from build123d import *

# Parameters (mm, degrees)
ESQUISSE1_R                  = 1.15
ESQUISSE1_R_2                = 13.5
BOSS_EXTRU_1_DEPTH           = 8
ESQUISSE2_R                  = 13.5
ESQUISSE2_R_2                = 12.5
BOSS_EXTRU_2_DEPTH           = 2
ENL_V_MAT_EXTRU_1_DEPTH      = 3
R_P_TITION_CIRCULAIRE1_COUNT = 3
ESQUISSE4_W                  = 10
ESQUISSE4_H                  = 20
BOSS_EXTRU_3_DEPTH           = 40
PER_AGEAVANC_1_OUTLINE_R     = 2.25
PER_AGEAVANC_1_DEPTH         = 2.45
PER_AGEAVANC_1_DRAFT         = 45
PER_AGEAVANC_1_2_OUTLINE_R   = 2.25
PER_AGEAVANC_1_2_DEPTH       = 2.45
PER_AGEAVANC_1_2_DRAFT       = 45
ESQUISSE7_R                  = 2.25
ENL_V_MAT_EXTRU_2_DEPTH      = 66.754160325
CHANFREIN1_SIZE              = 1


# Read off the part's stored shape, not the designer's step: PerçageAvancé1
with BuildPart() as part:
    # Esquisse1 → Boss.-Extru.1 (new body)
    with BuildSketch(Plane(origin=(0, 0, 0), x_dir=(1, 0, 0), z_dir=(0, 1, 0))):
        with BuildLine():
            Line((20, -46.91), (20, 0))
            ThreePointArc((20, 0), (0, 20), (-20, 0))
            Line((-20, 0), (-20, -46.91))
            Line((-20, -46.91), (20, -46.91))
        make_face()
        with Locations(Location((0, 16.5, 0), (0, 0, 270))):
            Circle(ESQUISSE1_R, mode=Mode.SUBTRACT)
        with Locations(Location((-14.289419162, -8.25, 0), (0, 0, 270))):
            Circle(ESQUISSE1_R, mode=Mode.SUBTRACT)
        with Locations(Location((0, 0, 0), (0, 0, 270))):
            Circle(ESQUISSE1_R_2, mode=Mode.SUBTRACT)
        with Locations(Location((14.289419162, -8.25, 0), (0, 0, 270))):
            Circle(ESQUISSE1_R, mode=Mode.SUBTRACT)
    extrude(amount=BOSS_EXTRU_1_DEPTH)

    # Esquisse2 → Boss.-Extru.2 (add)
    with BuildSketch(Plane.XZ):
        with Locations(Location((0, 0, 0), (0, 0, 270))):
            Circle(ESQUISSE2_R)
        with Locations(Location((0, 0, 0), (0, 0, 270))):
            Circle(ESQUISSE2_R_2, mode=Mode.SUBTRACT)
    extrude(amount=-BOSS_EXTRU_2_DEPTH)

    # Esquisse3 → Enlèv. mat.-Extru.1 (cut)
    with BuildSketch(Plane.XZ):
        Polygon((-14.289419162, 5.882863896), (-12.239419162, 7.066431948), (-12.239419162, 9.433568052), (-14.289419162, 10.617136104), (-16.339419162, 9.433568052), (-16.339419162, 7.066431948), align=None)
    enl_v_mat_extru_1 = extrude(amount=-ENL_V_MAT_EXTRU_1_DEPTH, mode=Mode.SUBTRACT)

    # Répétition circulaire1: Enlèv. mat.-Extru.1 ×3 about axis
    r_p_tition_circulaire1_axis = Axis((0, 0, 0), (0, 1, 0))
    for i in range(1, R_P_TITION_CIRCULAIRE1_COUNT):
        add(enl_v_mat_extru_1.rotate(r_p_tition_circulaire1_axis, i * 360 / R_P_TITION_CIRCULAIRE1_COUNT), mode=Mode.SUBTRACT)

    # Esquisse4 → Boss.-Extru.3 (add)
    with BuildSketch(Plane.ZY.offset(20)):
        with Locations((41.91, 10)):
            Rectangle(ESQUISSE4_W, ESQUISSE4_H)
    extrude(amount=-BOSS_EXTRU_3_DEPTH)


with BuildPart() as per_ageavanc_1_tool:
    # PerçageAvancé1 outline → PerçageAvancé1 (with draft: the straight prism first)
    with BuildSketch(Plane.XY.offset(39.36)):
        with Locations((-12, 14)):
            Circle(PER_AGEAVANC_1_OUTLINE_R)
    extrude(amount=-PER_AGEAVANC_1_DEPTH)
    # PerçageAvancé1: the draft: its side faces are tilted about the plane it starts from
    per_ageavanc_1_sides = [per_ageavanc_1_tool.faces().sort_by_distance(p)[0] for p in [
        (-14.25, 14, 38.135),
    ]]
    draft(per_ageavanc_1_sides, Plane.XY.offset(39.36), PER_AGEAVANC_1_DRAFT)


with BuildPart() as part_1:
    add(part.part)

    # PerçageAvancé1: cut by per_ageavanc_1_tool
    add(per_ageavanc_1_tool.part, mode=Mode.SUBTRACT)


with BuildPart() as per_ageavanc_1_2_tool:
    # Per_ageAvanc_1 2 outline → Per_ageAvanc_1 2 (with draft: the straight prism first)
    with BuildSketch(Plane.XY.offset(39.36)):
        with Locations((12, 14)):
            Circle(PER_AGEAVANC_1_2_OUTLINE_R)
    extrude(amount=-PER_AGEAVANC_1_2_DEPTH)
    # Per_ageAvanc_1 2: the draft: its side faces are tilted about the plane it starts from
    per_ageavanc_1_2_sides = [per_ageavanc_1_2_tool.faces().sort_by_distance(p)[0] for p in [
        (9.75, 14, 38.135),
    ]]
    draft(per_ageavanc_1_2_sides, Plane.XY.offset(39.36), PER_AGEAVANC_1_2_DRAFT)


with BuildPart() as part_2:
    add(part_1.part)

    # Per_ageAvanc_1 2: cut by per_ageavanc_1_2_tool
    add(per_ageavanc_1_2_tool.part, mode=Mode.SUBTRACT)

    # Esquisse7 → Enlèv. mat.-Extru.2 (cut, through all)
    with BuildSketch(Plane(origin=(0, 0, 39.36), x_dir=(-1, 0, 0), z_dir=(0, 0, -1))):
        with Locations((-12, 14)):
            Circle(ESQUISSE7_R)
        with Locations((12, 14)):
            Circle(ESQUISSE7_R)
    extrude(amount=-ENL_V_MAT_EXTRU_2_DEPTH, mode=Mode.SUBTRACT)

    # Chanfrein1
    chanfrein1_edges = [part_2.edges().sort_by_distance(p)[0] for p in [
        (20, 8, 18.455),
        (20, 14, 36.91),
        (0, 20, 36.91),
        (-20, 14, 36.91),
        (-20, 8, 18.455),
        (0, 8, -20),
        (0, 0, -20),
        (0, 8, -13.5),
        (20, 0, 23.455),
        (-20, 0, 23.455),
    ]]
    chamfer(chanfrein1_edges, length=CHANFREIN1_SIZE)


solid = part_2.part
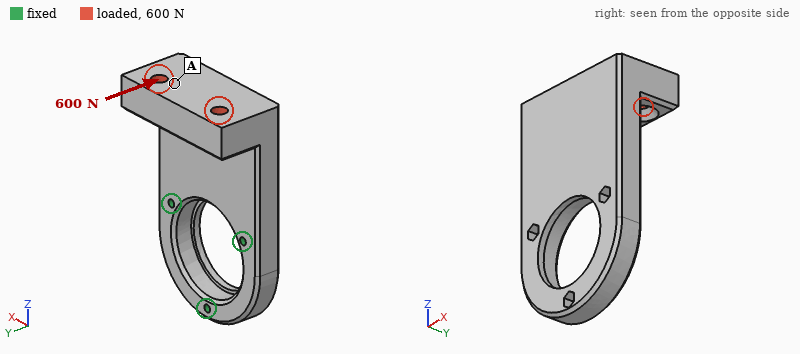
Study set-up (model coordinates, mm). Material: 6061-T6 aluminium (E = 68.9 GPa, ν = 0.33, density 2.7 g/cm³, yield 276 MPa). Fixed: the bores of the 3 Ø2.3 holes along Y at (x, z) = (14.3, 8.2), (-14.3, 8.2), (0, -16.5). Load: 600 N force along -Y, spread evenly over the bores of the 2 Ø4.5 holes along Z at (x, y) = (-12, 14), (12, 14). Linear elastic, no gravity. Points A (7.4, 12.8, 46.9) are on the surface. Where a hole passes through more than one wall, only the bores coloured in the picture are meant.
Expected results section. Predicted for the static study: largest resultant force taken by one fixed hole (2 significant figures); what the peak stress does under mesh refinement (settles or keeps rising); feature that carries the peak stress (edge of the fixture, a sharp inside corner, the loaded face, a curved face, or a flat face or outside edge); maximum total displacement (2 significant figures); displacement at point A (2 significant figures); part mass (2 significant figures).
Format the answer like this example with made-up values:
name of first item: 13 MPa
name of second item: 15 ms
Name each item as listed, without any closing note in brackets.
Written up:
largest resultant force taken by one fixed hole: 430 N
what the peak stress does under mesh refinement: keeps rising
feature that carries the peak stress: edge of the fixture
maximum total displacement: 0.23 mm
displacement at point A: 0.22 mm
part mass: 53 g
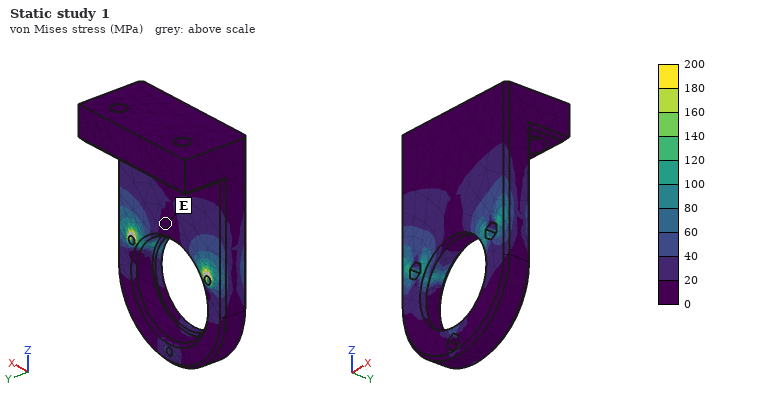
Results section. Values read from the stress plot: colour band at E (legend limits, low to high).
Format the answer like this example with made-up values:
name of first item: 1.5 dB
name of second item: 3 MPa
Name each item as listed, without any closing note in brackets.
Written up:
colour band at E: 0 to 20 MPa
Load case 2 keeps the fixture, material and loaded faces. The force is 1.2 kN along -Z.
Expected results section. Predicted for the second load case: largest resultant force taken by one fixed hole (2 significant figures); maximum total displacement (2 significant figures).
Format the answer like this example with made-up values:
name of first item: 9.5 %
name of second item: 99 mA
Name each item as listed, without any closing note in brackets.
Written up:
largest resultant force taken by one fixed hole: 640 N
maximum total displacement: 0.16 mm
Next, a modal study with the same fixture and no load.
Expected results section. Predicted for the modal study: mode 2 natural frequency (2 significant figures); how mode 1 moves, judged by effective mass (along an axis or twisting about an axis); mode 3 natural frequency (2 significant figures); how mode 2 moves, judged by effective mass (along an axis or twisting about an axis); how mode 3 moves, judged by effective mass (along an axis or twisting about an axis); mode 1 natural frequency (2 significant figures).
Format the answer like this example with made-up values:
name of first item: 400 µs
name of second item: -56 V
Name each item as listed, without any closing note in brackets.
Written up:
mode 2 natural frequency: 5300 Hz
how mode 1 moves, judged by effective mass: along Y
mode 3 natural frequency: 9100 Hz
how mode 2 moves, judged by effective mass: along X
how mode 3 moves, judged by effective mass: along X
mode 1 natural frequency: 1800 Hz
